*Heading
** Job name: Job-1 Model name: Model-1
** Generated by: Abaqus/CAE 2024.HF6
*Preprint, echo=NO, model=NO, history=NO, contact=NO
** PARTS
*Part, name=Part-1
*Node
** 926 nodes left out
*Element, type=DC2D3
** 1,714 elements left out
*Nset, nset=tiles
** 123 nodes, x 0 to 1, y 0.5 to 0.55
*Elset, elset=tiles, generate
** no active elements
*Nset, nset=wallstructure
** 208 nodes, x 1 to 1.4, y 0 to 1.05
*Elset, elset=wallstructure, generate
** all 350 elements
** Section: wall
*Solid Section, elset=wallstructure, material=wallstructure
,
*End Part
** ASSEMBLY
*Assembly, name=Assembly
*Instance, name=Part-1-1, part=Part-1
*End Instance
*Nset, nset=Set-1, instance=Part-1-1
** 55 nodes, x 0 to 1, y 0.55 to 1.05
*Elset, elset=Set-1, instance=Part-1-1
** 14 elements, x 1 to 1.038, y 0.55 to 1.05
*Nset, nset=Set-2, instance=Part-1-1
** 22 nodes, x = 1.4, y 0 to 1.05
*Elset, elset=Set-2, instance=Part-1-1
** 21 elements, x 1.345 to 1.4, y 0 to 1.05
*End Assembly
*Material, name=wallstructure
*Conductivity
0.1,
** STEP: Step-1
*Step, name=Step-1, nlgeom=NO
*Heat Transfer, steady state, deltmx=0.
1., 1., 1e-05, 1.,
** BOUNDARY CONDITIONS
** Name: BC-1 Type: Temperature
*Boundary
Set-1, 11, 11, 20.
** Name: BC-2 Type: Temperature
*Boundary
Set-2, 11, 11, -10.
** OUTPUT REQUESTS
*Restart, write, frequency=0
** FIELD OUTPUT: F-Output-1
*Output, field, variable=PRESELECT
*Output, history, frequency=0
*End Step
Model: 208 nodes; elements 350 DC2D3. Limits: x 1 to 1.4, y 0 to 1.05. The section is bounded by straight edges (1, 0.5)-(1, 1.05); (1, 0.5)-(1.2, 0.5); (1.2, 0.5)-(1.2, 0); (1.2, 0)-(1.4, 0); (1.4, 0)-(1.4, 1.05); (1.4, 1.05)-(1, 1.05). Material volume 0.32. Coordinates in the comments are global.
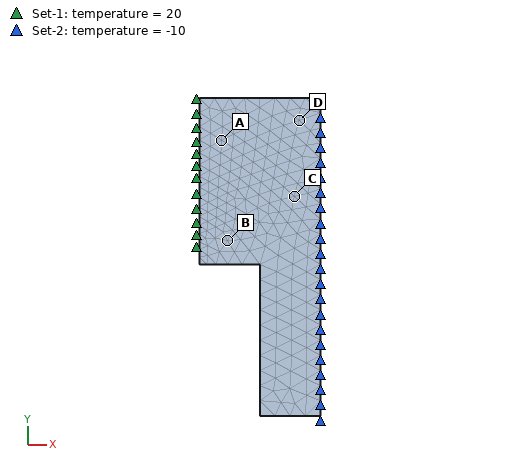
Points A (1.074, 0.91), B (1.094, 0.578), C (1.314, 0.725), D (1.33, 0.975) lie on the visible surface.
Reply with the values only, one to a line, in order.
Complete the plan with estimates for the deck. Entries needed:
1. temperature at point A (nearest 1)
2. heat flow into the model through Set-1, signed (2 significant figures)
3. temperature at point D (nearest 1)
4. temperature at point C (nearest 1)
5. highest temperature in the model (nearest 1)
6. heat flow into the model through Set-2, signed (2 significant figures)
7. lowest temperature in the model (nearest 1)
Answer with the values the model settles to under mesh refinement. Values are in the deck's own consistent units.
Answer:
14
4.3
-5
-4
20
-4.3
-10
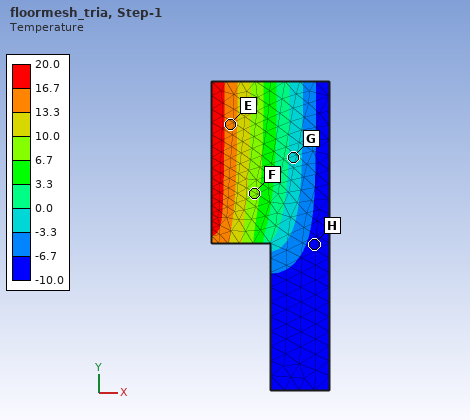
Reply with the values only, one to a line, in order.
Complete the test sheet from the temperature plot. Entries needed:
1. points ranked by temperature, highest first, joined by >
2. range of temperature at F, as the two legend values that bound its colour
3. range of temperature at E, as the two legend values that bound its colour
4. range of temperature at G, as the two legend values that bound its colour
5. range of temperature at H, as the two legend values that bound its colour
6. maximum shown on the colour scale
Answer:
E > F > G > H
6.7 to 10.0
13.3 to 16.7
-3.3 to 0.0
-10.0 to -6.7
20.0
